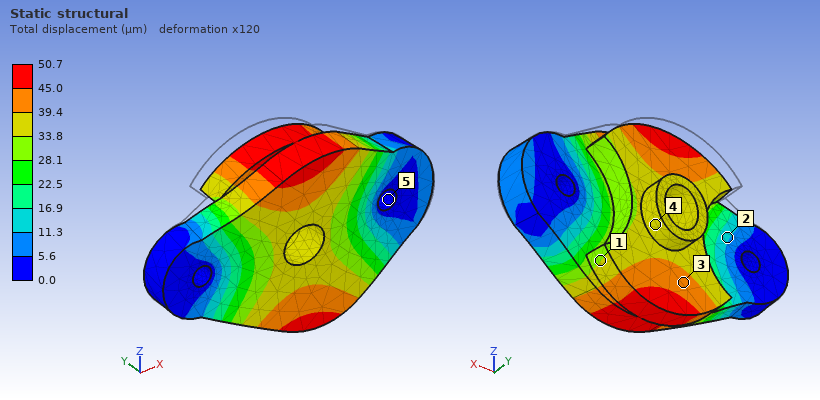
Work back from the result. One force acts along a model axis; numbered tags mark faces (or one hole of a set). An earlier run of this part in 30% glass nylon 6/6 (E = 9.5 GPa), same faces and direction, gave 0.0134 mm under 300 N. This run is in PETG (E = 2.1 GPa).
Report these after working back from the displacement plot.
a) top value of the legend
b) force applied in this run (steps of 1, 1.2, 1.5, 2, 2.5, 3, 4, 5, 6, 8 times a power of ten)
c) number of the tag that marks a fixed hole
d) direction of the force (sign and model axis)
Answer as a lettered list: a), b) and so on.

a) 50.7 µm
b) 250 N
c) 5
d) -Y
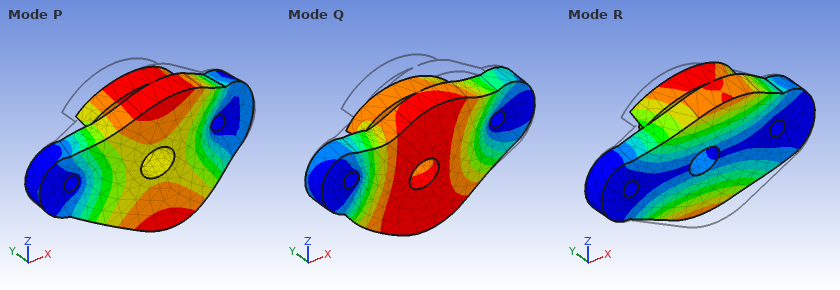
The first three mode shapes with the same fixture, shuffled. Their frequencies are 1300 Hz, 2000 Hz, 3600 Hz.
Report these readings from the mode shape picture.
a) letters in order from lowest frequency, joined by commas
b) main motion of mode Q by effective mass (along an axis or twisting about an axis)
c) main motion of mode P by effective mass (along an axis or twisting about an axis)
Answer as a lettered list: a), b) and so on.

a) R, P, Q
b) along Z
c) along Y
